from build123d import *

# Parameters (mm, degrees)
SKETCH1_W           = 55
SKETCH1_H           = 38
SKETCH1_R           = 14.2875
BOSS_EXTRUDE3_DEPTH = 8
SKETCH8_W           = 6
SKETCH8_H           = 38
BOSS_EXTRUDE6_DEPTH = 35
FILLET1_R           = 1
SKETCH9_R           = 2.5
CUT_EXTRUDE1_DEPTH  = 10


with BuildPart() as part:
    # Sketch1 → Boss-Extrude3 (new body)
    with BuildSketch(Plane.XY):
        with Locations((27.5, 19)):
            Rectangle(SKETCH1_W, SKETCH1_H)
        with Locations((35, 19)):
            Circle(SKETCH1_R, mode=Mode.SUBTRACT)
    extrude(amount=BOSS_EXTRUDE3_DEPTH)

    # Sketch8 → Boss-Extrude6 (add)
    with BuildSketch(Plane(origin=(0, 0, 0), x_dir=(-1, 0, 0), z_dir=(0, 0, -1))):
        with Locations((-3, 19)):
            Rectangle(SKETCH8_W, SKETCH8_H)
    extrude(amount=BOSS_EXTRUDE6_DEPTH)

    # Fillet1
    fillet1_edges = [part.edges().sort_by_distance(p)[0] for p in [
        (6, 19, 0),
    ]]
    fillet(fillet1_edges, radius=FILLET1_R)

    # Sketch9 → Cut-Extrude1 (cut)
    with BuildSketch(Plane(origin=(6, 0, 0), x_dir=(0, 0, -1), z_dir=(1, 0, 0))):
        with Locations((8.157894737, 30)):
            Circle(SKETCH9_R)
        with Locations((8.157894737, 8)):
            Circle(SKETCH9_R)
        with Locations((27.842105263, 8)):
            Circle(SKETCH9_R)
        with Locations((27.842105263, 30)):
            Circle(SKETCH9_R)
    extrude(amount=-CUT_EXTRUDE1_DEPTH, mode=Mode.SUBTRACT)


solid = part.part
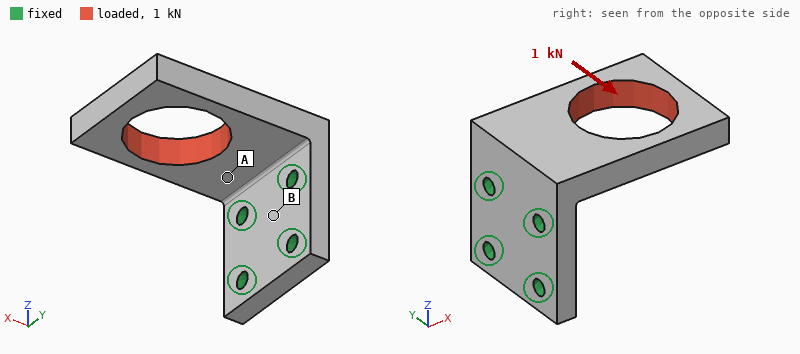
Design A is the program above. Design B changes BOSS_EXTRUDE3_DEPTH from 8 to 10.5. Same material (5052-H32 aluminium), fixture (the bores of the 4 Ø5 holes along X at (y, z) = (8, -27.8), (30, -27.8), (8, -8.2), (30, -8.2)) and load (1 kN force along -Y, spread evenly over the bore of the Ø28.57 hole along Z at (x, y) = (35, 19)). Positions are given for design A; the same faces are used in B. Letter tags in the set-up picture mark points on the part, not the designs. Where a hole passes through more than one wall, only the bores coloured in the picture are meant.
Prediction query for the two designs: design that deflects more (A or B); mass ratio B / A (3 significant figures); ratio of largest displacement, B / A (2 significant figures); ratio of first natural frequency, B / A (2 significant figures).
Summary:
A
1.19
0.86
0.98
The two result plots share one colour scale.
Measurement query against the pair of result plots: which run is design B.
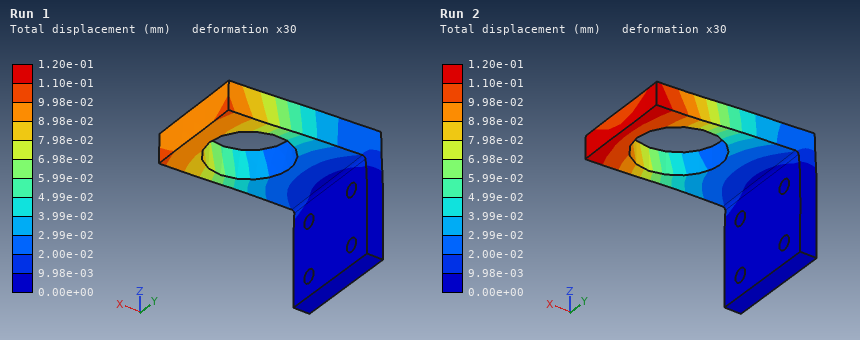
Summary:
Run 1
